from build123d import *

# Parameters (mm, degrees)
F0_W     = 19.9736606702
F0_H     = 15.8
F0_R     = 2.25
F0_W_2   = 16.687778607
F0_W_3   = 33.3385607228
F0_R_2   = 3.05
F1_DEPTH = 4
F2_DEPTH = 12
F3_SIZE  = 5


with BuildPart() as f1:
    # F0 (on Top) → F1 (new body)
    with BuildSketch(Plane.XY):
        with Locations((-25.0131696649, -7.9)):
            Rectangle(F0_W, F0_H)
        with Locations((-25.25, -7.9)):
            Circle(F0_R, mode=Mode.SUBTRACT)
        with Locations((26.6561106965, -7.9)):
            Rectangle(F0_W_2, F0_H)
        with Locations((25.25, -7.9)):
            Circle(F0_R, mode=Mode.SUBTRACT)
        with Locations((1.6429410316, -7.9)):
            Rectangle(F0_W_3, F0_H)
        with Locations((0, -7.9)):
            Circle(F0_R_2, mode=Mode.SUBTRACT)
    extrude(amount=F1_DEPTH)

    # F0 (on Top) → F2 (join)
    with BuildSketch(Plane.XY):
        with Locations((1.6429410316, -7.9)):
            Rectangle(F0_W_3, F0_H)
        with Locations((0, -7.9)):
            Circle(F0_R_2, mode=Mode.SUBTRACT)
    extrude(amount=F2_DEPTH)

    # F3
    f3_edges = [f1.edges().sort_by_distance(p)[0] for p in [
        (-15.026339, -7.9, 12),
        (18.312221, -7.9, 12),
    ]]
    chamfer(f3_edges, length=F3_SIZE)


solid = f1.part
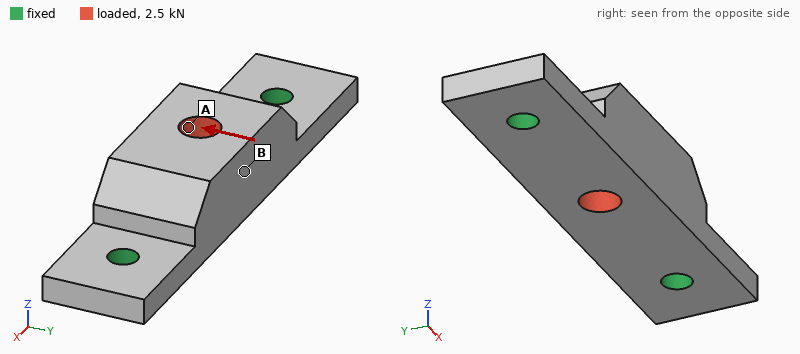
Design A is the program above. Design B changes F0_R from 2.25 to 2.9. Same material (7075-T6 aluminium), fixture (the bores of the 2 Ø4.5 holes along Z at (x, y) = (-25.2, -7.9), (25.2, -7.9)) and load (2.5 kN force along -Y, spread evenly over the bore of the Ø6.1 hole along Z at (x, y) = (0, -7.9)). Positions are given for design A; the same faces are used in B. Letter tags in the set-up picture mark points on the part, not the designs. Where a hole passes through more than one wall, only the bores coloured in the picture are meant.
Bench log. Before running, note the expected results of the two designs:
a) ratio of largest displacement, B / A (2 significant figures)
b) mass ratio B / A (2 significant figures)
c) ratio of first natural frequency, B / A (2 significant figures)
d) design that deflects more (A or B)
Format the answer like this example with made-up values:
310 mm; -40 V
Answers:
0.84; 0.99; 1.1; A
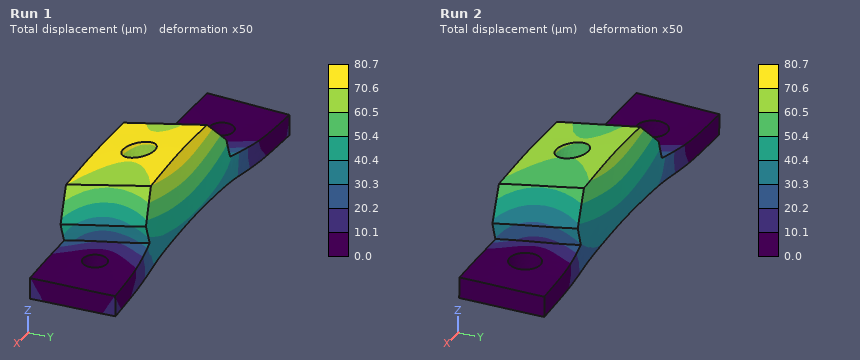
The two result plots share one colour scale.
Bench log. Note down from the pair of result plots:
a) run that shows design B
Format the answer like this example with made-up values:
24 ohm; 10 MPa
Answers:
Run 2
